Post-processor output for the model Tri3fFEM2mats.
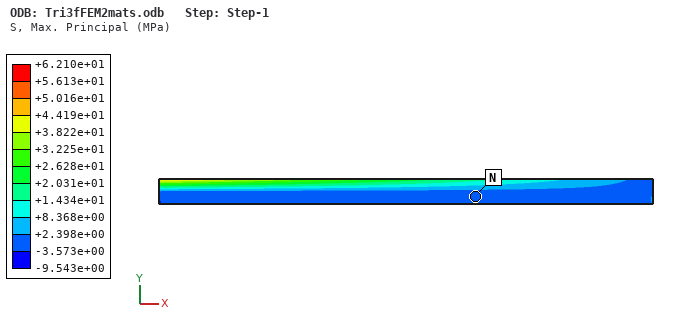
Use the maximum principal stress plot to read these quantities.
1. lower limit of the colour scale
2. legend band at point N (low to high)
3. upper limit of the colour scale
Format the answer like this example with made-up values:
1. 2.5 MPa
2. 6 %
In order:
1. -9.543e+00 MPa
2. -3.573e+00 to +2.398e+00 MPa
3. +6.210e+01 MPa
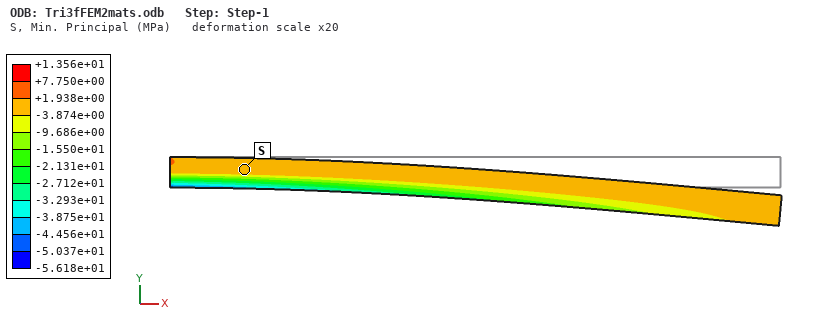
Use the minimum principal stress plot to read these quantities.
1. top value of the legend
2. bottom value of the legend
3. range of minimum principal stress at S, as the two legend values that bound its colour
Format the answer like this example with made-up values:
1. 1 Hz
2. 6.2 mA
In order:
1. +1.356e+01 MPa
2. -5.618e+01 MPa
3. -3.874e+00 to +1.938e+00 MPa
